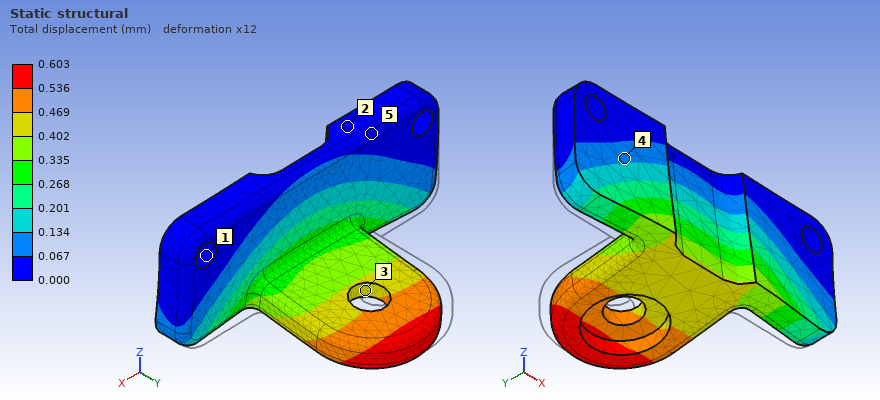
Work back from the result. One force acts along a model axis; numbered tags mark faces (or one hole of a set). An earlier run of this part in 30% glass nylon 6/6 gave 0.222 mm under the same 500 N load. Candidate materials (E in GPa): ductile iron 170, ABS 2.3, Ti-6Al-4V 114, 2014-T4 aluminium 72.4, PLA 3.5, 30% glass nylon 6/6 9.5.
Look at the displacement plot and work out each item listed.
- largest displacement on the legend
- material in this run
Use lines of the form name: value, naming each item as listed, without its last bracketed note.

largest displacement on the legend: 0.603 mm
material in this run: PLA
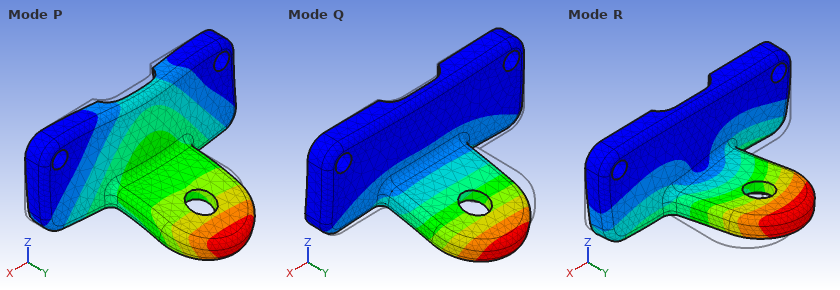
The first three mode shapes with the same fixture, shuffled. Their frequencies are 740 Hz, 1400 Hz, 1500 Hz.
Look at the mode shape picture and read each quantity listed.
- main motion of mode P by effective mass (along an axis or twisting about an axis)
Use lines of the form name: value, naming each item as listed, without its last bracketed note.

main motion of mode P by effective mass: along Y
